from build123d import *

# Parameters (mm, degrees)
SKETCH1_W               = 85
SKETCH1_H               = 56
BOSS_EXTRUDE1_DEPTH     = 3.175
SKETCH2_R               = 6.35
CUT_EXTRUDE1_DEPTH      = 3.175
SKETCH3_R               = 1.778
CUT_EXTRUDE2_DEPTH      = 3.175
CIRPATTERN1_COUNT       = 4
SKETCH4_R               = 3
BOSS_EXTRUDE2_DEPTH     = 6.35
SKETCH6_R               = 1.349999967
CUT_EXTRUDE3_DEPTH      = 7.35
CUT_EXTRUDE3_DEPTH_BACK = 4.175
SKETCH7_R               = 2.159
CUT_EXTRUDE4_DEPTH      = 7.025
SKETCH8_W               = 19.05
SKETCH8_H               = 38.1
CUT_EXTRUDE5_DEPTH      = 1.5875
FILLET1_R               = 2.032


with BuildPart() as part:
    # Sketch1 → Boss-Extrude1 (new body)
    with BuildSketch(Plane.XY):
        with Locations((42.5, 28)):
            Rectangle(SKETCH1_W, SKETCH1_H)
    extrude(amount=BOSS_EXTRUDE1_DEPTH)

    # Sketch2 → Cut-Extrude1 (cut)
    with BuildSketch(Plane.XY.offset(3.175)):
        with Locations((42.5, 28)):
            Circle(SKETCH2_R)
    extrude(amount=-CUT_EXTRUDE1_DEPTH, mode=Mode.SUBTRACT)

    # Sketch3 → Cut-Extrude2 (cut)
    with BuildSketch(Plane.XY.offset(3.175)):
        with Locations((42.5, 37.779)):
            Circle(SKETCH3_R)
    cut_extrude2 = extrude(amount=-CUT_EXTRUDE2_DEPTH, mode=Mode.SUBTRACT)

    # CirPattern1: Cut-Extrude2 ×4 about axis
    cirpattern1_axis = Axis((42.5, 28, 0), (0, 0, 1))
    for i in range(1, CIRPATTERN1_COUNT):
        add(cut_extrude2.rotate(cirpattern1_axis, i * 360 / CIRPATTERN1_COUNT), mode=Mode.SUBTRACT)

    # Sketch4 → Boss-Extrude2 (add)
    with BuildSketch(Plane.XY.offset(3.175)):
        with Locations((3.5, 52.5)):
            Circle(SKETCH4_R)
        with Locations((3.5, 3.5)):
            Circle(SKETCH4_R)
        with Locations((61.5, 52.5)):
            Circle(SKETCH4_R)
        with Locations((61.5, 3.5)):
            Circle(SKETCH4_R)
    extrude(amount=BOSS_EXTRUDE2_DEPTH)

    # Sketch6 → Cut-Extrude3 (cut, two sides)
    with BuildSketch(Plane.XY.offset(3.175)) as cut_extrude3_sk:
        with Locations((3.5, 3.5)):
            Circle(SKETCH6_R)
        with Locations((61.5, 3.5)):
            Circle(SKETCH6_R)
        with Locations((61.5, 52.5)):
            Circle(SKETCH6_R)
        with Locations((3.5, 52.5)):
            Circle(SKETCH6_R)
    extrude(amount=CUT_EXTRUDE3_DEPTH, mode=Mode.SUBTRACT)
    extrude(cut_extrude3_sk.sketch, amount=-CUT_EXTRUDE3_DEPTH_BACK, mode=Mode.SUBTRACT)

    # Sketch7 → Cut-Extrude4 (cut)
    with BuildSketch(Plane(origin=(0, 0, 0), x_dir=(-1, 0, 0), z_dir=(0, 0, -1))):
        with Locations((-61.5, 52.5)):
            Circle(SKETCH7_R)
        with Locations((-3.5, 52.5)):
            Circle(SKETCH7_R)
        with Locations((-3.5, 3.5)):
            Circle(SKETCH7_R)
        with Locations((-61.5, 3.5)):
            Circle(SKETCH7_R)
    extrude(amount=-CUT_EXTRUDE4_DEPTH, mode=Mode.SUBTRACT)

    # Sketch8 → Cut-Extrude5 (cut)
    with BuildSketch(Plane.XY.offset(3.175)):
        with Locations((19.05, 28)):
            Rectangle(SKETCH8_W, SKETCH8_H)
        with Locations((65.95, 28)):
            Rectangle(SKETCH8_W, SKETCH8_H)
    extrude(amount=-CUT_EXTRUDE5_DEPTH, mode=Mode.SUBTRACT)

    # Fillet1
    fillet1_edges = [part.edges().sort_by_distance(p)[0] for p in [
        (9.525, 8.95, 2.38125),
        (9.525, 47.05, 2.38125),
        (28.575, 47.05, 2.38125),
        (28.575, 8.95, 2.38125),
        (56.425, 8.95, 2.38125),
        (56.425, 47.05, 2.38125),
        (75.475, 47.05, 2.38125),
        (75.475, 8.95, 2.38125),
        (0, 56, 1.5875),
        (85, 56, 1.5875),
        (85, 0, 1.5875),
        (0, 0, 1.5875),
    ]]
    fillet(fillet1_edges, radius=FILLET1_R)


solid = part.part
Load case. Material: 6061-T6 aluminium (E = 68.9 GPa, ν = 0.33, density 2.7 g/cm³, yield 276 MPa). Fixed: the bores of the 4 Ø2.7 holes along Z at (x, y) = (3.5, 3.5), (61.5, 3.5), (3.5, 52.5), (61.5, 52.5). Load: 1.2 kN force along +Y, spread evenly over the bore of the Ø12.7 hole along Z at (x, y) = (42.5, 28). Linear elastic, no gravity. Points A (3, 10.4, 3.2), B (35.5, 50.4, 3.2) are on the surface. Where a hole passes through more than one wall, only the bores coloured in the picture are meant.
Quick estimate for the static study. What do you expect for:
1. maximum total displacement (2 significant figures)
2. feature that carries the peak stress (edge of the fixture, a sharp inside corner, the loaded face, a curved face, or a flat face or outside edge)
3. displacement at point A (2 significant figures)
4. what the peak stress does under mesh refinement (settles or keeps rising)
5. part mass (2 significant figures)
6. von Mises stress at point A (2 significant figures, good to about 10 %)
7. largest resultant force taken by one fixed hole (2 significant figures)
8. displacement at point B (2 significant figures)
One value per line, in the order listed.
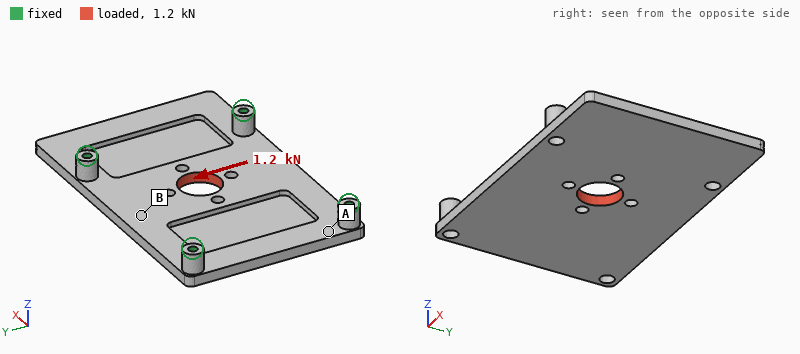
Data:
28 µm
edge of the fixture
15 µm
keeps rising
34 g
21 MPa
370 N
26 µm
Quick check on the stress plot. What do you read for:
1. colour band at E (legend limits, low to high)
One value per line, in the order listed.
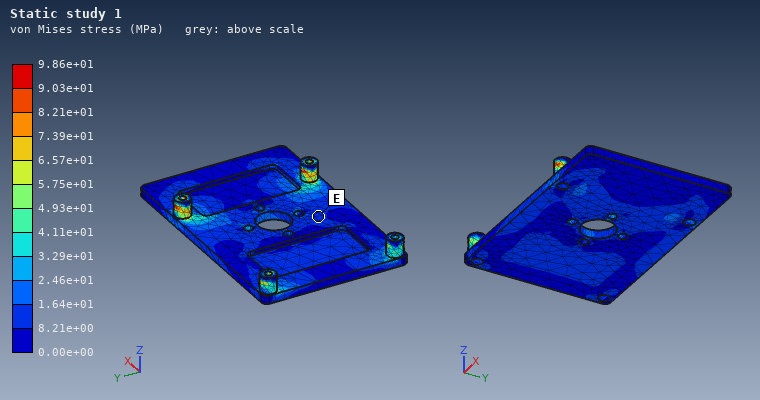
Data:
8.21e+00 to 1.64e+01 MPa
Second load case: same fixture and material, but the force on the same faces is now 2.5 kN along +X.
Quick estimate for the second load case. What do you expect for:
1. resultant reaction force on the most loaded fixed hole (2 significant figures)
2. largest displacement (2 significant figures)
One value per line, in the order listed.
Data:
670 N
0.12 mm
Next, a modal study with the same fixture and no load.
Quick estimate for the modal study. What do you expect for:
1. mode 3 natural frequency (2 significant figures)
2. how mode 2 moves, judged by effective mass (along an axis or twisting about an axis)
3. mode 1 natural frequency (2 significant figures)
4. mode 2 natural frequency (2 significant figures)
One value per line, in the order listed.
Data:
4500 Hz
along Z
2400 Hz
3100 Hz
